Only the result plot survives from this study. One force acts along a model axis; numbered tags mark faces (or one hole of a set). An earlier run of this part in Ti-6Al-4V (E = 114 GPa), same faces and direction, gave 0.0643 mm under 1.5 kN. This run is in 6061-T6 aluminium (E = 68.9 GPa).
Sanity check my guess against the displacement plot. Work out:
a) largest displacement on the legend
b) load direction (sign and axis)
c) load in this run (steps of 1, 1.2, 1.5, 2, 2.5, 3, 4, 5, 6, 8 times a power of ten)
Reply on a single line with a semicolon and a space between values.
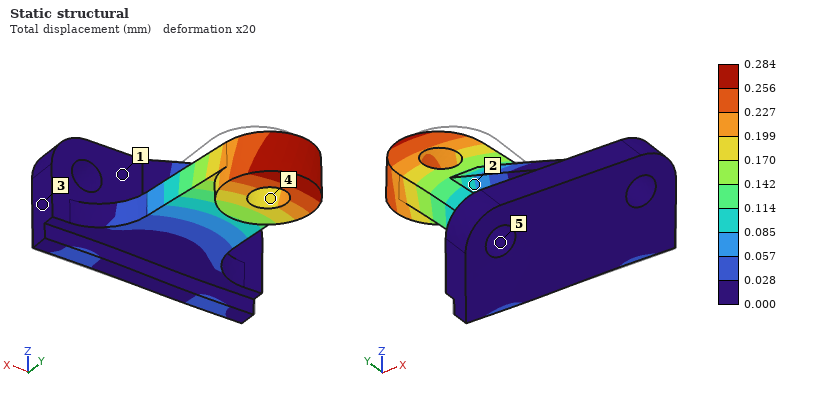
0.284 mm; -X; 4 kN
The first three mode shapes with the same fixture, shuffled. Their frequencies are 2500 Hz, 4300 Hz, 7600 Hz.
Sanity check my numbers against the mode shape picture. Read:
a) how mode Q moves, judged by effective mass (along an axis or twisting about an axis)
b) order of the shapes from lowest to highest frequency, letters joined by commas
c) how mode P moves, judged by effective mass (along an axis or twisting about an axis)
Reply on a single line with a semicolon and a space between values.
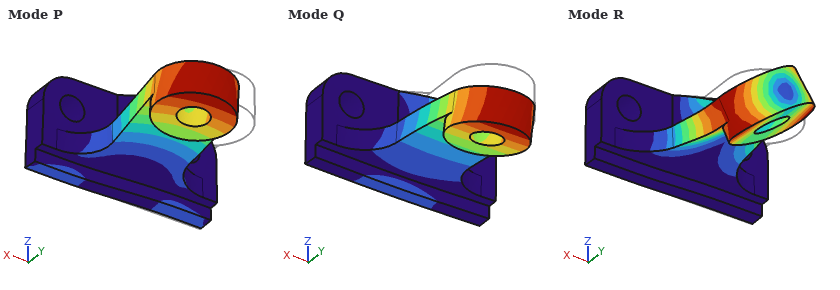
along Z; Q, P, R; along X
